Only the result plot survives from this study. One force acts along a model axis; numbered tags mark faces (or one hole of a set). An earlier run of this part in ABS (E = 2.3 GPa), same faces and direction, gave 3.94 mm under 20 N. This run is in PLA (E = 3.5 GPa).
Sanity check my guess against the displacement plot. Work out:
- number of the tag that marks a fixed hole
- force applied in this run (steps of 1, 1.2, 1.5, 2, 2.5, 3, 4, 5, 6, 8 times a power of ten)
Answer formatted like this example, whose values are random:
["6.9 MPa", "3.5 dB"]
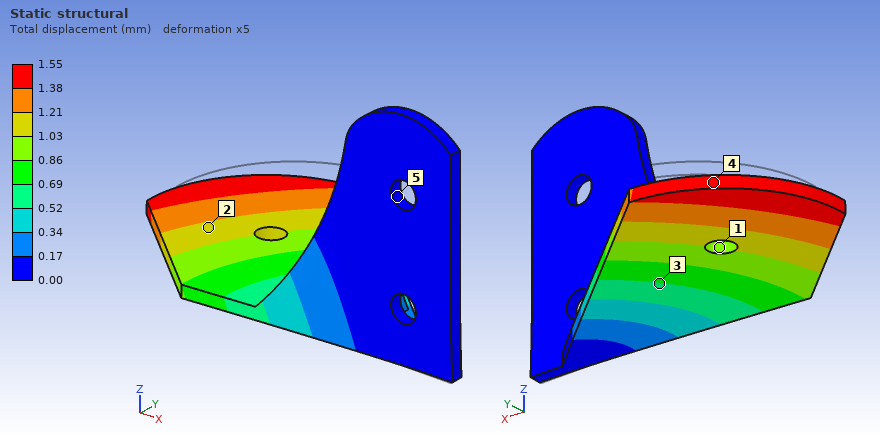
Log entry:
["5", "12 N"]
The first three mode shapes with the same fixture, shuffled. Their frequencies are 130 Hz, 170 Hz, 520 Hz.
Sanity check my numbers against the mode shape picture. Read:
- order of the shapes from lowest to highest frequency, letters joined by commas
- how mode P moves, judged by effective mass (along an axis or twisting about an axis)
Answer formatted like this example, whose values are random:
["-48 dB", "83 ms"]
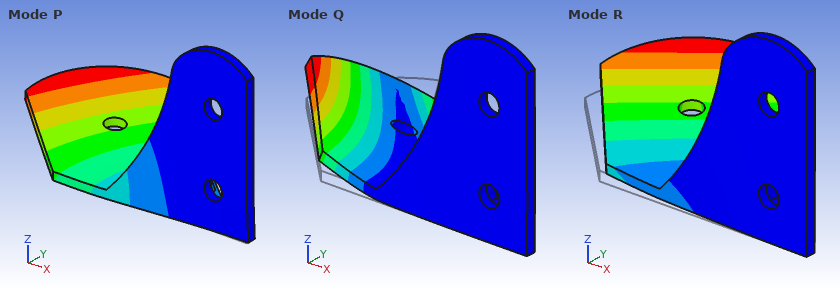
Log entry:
["R, P, Q", "along Y"]
